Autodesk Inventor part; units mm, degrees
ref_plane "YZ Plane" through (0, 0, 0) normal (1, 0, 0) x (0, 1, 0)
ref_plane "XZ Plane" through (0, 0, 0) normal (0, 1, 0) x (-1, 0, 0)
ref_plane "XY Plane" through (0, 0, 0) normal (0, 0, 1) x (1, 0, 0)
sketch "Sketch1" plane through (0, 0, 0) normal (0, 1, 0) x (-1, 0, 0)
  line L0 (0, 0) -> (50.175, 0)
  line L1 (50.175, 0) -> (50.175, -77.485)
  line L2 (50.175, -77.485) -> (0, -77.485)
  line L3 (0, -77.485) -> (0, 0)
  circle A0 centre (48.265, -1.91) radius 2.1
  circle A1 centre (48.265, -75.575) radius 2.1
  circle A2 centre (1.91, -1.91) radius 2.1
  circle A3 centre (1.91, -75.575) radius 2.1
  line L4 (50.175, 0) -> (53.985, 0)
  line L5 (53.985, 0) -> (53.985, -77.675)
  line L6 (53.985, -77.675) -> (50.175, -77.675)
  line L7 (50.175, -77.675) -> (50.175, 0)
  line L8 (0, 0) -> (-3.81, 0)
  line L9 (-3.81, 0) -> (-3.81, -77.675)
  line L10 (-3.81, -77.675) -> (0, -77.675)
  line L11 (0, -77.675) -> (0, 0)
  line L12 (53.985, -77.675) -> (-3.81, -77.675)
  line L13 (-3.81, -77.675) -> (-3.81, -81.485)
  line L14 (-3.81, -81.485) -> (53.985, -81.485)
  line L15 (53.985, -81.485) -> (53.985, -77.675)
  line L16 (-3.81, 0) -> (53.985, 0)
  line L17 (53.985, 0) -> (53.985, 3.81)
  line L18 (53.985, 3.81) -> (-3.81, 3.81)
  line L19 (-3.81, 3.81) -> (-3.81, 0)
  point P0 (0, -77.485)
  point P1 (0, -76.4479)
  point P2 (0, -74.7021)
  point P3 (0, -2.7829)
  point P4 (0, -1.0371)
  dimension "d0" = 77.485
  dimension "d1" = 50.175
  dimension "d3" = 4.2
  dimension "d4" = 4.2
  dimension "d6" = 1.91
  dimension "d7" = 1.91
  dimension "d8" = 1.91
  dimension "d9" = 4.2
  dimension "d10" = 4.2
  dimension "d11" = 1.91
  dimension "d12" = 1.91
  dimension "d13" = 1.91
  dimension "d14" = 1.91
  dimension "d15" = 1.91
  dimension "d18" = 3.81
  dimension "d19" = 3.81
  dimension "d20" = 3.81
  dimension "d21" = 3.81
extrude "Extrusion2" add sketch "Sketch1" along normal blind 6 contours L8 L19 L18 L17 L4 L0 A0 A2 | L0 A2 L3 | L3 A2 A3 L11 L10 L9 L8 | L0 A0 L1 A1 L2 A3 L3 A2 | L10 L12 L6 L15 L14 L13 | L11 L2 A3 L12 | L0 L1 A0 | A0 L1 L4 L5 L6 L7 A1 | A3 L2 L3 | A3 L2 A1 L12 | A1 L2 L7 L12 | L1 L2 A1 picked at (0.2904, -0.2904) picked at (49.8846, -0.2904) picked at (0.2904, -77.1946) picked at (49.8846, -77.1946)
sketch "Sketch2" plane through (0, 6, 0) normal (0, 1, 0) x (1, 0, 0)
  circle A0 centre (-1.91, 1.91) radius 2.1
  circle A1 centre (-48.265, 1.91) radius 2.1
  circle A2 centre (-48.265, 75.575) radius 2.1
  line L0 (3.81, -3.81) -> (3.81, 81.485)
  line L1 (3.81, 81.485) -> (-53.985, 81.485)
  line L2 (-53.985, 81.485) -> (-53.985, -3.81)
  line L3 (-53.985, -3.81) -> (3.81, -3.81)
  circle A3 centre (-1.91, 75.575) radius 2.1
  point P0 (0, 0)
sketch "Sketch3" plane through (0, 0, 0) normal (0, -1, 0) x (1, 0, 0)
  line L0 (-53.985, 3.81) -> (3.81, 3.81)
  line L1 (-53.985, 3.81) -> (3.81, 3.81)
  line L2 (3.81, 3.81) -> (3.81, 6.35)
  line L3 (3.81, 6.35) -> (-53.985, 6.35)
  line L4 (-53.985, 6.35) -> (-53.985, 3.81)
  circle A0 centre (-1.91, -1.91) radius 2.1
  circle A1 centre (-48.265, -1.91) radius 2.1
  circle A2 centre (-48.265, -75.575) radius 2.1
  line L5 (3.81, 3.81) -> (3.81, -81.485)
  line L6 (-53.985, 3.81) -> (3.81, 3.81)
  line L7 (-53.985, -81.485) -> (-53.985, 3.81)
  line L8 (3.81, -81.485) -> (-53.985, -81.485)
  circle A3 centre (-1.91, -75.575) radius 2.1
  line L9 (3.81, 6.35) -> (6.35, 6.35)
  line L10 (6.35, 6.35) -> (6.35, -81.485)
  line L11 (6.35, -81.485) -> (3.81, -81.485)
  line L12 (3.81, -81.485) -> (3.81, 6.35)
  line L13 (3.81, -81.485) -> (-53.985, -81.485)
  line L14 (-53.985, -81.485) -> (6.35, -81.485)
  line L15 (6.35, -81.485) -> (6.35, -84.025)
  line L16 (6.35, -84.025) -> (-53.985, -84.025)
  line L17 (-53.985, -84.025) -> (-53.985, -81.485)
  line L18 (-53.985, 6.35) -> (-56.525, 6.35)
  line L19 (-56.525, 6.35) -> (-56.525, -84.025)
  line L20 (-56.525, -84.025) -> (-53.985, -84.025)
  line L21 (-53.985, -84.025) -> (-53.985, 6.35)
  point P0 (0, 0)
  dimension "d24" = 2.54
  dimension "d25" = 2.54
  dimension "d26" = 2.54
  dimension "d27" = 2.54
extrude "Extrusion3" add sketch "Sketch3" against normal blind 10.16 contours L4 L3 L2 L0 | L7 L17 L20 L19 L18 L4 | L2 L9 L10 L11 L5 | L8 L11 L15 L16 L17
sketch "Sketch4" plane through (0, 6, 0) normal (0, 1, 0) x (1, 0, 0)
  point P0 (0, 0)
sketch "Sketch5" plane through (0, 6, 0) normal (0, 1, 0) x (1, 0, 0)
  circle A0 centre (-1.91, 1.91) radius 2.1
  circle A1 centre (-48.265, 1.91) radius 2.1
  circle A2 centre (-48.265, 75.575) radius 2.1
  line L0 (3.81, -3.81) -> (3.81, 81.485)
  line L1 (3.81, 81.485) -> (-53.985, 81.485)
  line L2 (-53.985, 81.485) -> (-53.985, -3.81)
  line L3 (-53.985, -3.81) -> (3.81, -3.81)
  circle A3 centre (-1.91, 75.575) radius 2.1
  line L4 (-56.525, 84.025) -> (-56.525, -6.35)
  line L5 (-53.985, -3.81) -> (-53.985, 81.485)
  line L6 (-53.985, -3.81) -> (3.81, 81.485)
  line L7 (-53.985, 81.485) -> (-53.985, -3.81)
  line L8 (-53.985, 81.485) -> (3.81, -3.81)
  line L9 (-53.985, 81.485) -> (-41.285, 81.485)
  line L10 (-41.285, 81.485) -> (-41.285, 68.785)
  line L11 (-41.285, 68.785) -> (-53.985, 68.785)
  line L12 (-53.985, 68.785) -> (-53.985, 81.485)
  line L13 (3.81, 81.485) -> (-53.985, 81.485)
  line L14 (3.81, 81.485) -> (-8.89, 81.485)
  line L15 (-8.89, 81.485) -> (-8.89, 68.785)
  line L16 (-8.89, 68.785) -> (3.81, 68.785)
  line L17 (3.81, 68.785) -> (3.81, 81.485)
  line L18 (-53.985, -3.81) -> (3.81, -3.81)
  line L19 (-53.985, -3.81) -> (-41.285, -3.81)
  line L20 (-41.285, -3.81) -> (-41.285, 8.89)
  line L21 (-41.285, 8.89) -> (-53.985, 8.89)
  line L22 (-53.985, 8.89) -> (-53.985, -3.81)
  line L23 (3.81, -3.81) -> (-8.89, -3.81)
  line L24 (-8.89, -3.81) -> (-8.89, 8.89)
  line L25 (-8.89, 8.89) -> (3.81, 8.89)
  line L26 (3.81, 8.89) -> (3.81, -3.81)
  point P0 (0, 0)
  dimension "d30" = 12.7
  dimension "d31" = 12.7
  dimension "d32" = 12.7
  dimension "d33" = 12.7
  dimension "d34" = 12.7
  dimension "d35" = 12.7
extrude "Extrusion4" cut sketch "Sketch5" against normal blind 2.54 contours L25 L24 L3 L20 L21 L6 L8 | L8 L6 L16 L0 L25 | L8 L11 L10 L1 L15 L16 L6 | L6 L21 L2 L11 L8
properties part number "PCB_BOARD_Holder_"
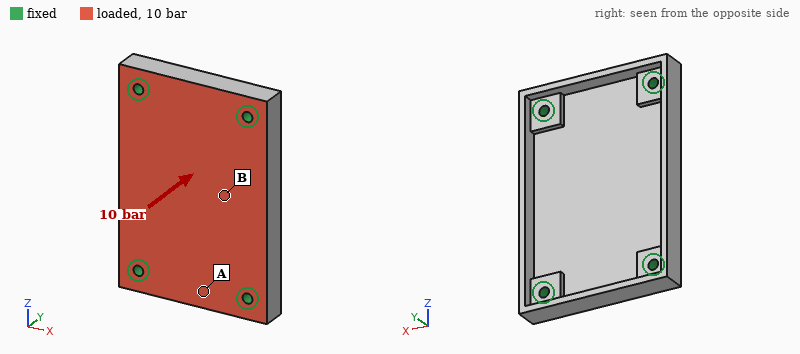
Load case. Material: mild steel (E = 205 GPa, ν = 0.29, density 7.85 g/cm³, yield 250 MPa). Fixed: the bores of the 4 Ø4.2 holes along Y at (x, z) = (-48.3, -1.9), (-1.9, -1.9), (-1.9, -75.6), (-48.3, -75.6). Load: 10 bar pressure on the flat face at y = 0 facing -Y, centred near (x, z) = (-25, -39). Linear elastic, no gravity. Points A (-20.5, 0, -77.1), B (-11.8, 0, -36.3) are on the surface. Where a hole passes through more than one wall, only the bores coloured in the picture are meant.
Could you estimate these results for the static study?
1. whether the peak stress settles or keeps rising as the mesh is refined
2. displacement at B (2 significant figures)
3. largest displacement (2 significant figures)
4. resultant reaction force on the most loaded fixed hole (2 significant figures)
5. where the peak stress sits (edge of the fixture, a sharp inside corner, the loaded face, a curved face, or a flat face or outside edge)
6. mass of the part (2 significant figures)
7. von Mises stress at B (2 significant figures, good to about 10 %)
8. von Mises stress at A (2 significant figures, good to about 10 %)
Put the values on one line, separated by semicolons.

keeps rising; 60 µm; 71 µm; 1.5 kN; edge of the fixture; 200 g; 65 MPa; 37 MPa
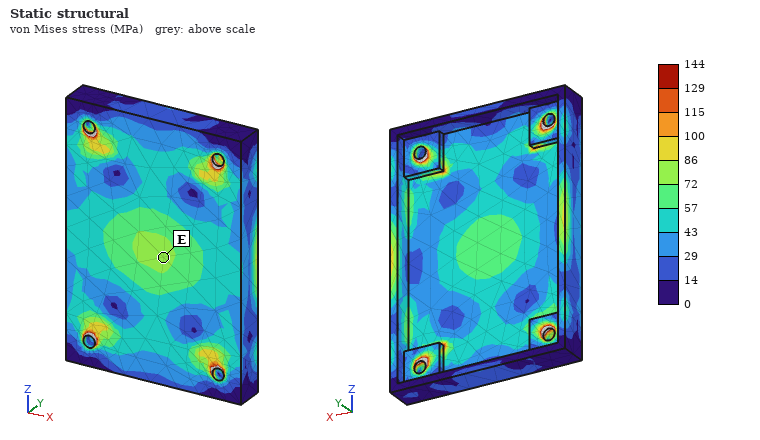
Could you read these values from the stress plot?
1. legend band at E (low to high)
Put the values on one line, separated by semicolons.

72 to 86 MPa
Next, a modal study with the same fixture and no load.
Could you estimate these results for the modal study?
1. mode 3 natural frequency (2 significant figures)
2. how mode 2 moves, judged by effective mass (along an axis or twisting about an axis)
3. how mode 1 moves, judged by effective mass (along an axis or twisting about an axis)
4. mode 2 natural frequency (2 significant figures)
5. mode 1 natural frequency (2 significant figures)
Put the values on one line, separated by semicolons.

8400 Hz; twisting about Z; along Y; 6800 Hz; 4500 Hz
